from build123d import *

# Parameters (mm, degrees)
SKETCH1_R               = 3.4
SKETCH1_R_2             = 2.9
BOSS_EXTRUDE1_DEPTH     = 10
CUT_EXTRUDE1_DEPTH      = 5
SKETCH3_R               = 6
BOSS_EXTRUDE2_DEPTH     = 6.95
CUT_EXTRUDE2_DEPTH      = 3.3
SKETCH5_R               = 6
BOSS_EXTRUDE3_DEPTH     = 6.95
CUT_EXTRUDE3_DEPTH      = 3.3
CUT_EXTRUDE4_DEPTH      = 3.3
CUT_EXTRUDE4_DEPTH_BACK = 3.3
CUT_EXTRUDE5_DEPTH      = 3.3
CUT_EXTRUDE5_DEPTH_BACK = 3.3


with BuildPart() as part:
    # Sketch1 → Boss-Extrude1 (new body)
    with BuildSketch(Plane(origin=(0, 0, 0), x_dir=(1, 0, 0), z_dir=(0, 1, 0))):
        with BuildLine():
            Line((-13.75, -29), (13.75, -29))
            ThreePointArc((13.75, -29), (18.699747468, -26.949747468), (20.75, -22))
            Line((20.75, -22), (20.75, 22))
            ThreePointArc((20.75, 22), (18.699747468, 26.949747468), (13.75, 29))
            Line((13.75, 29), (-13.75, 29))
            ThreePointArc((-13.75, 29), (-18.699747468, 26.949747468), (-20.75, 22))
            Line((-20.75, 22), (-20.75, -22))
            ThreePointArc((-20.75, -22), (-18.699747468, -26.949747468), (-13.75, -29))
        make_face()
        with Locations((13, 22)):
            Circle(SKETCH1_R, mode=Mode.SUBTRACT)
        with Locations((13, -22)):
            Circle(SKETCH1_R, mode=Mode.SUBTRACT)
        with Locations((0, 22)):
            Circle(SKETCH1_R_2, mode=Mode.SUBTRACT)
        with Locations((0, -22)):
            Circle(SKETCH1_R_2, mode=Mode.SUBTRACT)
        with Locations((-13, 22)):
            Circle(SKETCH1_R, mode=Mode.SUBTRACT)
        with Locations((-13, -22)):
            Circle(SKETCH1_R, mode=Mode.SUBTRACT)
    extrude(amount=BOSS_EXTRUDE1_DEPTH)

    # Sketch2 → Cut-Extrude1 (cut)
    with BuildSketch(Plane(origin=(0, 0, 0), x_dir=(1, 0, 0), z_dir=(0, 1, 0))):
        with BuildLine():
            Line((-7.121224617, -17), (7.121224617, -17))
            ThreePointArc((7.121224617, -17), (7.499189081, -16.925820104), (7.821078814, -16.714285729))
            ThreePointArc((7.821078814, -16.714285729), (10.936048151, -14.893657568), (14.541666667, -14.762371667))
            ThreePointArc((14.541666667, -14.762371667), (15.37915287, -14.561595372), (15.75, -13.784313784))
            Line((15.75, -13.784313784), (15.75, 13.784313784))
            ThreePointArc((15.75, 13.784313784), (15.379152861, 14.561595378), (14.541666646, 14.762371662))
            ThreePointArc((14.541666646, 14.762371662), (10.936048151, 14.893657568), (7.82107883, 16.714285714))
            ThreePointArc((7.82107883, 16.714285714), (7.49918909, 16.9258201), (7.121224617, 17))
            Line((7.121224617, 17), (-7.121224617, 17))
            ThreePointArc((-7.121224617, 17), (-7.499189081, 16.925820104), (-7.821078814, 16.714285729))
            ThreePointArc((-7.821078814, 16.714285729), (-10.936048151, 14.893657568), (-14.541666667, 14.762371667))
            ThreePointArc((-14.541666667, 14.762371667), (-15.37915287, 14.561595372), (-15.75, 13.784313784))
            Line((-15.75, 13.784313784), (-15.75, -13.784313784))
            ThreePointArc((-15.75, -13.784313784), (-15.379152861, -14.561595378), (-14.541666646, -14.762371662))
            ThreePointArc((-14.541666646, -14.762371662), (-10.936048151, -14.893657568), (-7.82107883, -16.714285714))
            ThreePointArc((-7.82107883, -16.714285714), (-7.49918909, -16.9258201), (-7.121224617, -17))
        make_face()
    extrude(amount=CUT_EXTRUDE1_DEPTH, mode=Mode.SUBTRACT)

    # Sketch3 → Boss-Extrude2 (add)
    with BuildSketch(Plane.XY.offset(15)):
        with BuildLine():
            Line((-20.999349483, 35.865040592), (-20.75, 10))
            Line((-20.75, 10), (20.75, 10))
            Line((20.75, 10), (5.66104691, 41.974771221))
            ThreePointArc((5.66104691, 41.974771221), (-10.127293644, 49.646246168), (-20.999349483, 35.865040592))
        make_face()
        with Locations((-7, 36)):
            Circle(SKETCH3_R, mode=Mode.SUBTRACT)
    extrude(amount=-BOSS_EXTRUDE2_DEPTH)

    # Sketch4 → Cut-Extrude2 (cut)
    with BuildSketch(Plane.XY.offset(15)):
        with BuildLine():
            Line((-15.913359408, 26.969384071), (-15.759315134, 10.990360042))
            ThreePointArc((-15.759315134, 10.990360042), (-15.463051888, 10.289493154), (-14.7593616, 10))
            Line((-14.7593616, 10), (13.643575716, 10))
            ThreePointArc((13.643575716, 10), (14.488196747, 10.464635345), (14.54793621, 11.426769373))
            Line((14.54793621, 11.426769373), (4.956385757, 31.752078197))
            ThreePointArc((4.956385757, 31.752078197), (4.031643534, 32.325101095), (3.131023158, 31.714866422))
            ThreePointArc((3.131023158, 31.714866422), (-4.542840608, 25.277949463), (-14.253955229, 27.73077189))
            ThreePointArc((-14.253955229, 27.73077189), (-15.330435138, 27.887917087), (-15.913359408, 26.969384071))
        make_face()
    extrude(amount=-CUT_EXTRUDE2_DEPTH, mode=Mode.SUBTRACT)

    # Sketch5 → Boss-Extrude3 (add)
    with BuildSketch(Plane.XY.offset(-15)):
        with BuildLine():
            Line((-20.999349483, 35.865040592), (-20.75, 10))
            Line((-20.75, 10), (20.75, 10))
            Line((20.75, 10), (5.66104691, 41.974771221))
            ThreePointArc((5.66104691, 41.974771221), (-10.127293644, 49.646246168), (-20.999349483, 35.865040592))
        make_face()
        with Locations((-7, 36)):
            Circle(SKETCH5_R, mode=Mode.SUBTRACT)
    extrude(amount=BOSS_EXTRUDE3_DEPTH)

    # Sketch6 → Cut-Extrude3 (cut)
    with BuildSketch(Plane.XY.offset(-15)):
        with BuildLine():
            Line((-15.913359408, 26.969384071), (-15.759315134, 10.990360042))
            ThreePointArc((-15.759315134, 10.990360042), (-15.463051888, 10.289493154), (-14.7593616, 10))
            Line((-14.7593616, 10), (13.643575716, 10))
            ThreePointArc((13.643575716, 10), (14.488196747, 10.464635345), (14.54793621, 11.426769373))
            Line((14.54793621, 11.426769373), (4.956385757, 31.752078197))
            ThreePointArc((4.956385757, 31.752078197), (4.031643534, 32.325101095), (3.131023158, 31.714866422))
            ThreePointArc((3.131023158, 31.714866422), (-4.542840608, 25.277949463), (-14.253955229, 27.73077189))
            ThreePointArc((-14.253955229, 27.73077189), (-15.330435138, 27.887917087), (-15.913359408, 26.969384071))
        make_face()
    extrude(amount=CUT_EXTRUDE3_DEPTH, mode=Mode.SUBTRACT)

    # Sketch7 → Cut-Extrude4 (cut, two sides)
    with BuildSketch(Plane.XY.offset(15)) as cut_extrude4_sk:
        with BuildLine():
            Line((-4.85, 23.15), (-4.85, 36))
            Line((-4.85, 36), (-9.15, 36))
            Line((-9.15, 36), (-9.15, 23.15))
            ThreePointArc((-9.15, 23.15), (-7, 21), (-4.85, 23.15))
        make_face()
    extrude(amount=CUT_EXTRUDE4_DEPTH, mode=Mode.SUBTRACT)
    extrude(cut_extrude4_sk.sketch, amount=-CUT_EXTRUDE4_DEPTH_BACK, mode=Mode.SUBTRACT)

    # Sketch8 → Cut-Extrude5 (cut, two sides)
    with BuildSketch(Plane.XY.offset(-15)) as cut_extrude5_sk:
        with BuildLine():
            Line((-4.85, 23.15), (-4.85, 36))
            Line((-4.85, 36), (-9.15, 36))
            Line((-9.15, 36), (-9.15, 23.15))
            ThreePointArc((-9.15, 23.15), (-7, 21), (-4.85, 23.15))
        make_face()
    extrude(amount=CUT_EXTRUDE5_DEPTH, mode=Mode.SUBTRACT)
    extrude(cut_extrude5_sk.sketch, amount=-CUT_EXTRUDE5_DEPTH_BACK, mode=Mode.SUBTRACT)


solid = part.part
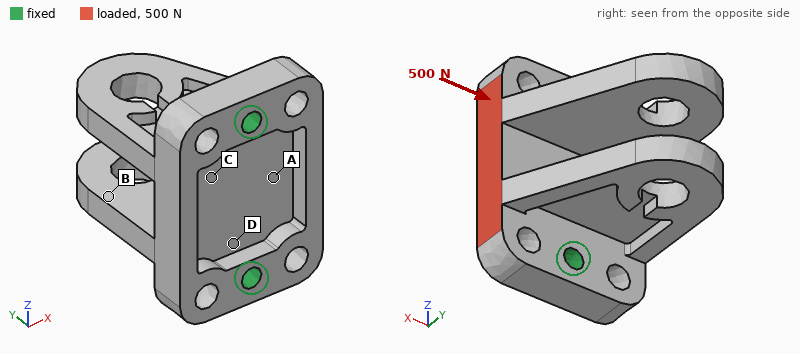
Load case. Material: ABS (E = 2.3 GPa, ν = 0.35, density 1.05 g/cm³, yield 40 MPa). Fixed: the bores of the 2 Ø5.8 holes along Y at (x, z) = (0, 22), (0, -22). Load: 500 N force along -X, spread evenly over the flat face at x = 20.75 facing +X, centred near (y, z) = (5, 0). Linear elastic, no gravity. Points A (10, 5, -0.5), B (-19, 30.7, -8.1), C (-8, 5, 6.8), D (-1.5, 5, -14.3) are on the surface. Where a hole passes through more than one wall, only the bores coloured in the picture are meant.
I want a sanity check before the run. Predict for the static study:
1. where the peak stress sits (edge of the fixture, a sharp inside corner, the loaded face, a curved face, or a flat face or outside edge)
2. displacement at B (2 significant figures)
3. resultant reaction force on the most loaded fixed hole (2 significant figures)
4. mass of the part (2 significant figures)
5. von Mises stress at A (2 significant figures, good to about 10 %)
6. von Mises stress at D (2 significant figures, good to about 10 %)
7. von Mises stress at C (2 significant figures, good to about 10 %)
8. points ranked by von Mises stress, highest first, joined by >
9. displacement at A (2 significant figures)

a curved face
22 µm
260 N
30 g
2.6 MPa
1.8 MPa
0.95 MPa
A > D > C > B
26 µm
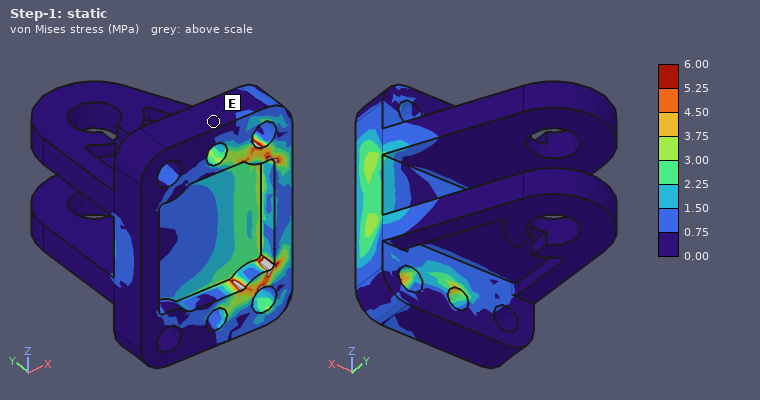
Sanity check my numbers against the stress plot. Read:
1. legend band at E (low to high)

0.00 to 0.75 MPa
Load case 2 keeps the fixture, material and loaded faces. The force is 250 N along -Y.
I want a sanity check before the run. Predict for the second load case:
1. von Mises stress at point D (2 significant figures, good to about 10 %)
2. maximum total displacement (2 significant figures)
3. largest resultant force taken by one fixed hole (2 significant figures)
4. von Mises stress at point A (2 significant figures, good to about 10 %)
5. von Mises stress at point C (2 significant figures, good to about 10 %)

2.6 MPa
0.24 mm
130 N
2.0 MPa
1.1 MPa
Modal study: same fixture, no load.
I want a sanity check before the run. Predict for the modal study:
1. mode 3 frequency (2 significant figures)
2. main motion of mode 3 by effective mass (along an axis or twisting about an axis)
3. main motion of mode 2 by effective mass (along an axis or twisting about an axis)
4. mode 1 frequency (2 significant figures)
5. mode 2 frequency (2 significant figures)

1300 Hz
along X
along Z
780 Hz
830 Hz
